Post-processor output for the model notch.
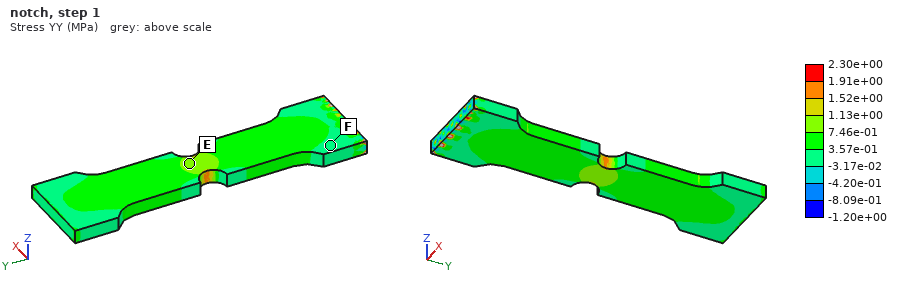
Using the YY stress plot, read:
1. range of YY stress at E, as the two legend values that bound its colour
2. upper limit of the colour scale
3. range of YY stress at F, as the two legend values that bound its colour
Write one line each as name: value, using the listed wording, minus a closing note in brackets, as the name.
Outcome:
range of YY stress at E, as the two legend values that bound its colour: 7.46e-01 to 1.13e+00 MPa
upper limit of the colour scale: 2.30e+00 MPa
range of YY stress at F, as the two legend values that bound its colour: -3.17e-02 to 3.57e-01 MPa
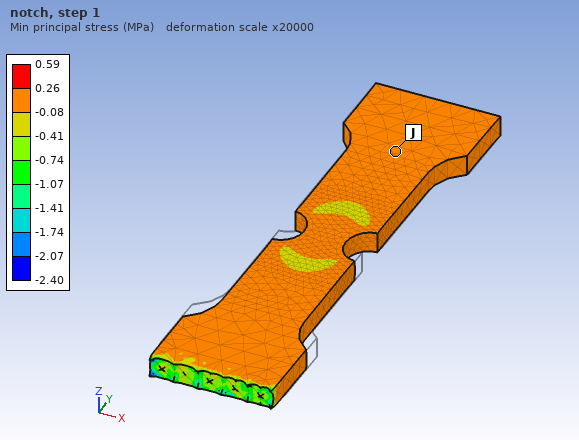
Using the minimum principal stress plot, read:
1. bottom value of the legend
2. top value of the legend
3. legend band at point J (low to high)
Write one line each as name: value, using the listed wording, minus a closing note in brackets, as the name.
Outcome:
bottom value of the legend: -2.40 MPa
top value of the legend: 0.59 MPa
legend band at point J: -0.08 to 0.26 MPa
